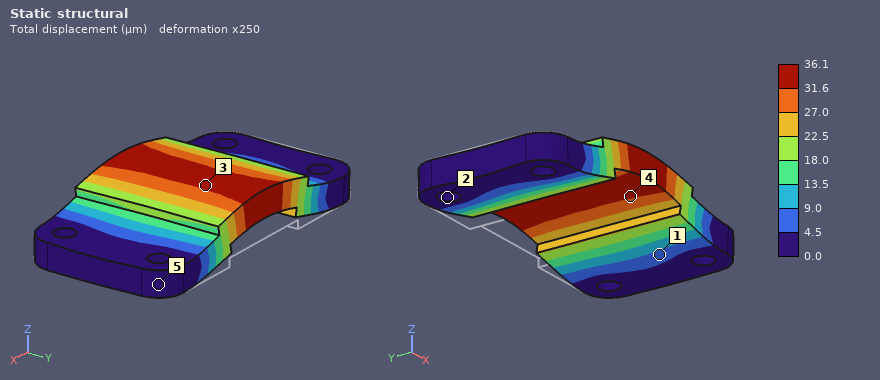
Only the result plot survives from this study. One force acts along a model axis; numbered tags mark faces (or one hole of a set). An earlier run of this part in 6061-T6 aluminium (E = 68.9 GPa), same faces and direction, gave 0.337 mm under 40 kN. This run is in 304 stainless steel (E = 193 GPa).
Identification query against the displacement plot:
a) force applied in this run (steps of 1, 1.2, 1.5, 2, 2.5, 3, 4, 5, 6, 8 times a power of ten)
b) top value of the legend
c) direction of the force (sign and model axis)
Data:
12 kN
36.1 µm
+Z
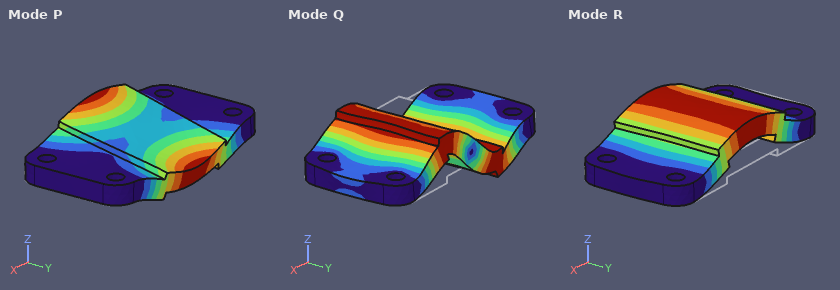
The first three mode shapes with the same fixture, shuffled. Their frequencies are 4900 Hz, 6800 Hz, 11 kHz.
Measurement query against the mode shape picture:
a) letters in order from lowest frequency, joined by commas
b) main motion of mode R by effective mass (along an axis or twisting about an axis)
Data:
R, P, Q
along Z
